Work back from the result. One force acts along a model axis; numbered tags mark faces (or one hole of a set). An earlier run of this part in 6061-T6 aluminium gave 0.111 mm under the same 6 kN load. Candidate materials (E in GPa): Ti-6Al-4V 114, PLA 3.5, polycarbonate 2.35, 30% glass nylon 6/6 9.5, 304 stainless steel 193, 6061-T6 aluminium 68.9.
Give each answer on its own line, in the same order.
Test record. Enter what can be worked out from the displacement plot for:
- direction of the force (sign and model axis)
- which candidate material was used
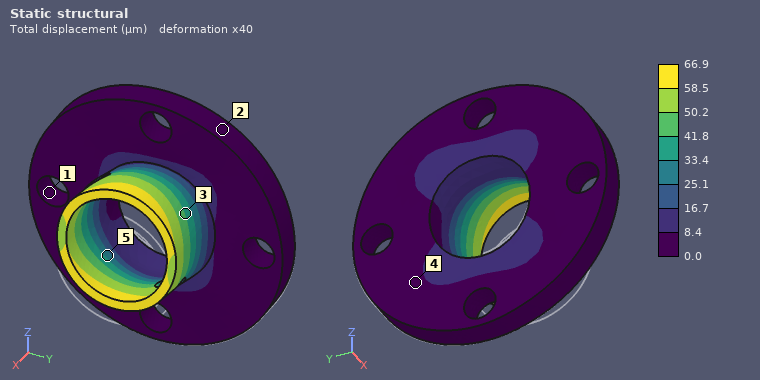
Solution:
+Z
Ti-6Al-4V
